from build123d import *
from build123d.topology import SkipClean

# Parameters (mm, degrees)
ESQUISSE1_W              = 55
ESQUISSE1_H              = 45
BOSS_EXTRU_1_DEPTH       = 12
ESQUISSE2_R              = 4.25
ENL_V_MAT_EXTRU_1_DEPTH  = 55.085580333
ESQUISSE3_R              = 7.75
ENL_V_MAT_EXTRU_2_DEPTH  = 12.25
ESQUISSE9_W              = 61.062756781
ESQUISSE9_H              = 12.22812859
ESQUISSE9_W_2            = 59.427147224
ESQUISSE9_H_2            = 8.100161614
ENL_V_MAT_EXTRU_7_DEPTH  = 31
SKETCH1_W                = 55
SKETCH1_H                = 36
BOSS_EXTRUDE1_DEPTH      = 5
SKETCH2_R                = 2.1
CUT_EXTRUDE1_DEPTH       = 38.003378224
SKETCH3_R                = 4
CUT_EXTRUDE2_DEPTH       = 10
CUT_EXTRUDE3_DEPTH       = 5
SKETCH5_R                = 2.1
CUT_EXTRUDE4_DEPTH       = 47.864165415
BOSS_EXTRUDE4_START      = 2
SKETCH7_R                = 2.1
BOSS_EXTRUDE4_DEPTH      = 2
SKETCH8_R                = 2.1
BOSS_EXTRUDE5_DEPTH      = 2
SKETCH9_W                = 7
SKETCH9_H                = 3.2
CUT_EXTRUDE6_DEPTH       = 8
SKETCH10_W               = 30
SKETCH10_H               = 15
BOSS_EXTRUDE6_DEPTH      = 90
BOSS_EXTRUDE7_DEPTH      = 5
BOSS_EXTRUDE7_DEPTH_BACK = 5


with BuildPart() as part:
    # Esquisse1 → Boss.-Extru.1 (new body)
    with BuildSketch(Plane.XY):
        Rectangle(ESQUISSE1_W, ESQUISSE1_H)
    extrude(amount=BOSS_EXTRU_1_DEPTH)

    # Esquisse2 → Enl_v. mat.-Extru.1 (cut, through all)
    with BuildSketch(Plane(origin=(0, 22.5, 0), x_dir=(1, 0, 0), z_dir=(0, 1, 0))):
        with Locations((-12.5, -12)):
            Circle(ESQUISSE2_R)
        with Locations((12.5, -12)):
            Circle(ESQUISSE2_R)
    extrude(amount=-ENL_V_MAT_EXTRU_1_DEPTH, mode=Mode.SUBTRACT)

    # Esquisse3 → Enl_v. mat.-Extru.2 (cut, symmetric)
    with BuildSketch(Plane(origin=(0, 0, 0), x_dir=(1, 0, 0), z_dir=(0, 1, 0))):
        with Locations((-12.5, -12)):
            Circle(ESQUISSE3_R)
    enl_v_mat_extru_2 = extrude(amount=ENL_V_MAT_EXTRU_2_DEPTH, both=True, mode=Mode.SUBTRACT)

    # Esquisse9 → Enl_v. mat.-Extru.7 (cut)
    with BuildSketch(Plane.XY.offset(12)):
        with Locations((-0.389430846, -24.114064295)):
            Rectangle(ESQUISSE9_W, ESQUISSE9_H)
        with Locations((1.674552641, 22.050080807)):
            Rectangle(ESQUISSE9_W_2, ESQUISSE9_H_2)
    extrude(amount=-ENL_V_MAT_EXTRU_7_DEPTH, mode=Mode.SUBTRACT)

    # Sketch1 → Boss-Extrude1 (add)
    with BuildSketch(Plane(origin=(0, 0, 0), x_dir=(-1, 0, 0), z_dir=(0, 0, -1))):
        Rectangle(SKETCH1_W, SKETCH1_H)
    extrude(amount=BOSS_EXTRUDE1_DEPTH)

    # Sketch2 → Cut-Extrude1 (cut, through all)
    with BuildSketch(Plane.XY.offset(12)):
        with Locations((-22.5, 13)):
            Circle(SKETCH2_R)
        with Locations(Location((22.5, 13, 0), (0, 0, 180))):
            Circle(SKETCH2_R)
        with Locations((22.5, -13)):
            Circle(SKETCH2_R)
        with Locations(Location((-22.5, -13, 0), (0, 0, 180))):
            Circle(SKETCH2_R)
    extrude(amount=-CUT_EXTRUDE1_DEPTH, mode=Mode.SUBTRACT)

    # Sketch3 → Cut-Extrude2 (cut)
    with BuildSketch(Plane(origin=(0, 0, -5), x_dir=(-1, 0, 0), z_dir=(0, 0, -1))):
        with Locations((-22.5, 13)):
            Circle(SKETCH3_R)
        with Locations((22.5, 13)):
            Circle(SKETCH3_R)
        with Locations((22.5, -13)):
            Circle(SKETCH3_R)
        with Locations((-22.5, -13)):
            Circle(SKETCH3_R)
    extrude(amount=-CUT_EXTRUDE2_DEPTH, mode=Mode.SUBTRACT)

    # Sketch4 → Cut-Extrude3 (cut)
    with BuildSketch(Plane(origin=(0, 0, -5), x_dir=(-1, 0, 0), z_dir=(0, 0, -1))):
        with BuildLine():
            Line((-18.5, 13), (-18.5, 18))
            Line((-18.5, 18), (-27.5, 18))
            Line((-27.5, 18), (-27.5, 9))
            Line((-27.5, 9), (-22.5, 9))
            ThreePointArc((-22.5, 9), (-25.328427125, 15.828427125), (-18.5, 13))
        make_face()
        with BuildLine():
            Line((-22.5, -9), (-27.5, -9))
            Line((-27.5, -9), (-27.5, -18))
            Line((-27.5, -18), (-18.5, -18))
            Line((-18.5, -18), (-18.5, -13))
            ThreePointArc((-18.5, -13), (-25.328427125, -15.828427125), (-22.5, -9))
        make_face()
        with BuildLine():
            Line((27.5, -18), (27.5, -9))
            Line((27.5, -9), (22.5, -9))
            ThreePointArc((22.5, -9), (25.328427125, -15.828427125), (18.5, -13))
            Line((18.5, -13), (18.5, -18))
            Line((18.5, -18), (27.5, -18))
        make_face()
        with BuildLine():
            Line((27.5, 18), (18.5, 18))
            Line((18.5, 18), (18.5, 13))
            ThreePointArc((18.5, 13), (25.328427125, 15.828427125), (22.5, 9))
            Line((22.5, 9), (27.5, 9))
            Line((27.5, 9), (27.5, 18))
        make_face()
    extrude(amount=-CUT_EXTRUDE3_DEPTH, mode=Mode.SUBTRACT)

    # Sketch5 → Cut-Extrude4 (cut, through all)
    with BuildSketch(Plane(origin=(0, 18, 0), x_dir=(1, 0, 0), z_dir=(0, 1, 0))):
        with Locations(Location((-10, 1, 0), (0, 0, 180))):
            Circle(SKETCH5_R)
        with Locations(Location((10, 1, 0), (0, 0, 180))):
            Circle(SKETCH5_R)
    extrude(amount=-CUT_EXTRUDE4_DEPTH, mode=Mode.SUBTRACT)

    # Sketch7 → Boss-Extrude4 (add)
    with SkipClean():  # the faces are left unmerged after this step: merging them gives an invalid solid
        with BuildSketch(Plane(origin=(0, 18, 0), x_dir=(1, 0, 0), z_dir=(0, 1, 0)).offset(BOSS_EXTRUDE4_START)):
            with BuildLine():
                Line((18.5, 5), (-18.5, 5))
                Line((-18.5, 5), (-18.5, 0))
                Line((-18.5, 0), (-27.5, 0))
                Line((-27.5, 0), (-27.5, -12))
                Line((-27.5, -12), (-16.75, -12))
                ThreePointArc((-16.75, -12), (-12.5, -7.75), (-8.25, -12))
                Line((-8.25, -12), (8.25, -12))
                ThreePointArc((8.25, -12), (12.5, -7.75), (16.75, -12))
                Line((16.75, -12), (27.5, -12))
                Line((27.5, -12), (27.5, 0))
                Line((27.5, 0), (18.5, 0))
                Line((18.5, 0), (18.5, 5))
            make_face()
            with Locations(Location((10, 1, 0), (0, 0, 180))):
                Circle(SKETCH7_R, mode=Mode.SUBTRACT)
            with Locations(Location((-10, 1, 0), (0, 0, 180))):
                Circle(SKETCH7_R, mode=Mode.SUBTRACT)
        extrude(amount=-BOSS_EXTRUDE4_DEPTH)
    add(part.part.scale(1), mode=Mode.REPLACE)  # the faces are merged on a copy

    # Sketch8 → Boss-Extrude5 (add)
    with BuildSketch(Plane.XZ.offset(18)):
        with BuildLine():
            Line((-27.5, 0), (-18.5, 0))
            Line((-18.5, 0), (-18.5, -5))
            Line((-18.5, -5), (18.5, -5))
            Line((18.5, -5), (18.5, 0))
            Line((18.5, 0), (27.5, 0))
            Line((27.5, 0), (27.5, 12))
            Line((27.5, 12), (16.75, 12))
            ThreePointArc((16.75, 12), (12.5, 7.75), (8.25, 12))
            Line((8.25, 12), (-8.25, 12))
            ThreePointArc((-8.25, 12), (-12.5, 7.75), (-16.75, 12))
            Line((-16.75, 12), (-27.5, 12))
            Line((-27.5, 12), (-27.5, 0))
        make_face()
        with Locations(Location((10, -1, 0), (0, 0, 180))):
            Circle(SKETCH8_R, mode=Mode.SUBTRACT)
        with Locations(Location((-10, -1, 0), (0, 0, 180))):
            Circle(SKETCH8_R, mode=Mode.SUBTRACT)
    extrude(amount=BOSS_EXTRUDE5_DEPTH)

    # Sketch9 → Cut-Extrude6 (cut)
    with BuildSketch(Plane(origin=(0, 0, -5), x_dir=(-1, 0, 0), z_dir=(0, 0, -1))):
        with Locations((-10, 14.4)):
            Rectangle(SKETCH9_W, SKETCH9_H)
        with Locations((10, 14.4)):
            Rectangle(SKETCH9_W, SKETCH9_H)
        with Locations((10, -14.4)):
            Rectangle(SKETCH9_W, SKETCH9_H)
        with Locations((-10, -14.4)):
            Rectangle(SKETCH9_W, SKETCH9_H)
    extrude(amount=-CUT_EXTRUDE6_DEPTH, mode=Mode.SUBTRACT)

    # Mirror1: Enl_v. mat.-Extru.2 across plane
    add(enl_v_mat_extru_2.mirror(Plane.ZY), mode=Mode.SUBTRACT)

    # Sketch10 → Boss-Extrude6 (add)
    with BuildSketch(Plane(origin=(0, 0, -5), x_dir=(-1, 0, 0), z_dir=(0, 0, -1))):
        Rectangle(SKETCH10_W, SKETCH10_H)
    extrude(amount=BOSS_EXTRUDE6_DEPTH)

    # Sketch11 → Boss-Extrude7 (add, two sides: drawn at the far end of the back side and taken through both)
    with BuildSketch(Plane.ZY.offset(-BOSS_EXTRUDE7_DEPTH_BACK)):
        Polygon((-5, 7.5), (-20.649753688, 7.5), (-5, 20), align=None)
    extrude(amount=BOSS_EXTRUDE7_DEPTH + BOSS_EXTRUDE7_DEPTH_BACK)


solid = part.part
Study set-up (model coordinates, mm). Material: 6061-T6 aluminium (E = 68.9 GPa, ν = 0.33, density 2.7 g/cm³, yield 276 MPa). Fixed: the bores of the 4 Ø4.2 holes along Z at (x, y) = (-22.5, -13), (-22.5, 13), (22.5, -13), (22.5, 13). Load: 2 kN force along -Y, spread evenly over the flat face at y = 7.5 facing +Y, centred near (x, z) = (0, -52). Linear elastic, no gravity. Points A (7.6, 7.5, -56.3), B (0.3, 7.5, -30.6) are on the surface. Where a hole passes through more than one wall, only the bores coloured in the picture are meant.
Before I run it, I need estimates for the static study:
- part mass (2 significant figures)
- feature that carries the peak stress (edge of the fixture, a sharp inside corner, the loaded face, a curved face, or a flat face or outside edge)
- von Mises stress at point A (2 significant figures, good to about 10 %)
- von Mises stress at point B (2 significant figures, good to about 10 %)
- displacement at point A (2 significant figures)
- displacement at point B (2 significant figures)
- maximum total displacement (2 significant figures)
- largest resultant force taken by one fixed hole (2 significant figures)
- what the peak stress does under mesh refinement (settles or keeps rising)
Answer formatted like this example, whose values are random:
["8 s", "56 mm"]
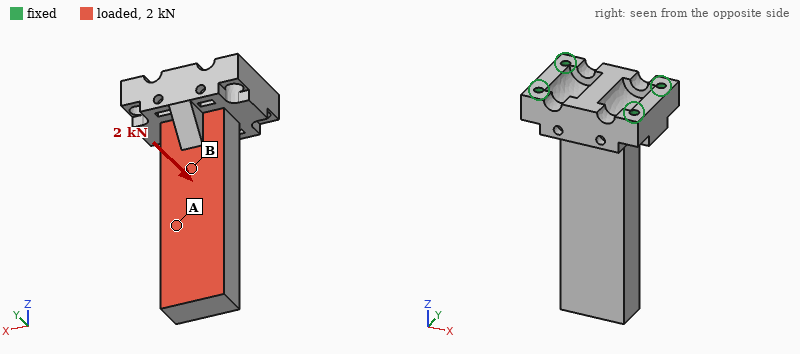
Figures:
["180 g", "edge of the fixture", "16 MPa", "45 MPa", "0.21 mm", "0.086 mm", "0.43 mm", "2.5 kN", "keeps rising"]
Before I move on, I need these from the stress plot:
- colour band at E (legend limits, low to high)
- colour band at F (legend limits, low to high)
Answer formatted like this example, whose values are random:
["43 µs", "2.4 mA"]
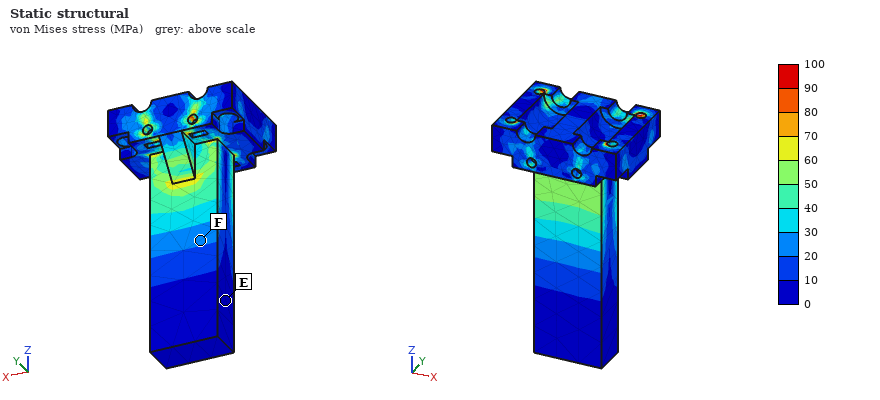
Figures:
["0 to 10 MPa", "20 to 30 MPa"]
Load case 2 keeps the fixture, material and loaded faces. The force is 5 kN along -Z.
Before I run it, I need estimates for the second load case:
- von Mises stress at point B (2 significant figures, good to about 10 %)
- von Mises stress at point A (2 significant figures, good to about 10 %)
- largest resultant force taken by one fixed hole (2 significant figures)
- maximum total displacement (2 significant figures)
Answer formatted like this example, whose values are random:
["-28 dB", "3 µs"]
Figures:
["35 MPa", "21 MPa", "2.2 kN", "0.21 mm"]
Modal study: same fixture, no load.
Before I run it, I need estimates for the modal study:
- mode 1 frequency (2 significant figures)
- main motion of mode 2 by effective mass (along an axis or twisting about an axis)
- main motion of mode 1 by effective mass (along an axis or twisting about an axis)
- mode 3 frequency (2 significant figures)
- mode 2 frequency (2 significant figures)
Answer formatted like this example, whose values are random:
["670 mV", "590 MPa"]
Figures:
["1300 Hz", "along X", "along Y", "6400 Hz", "2200 Hz"]
